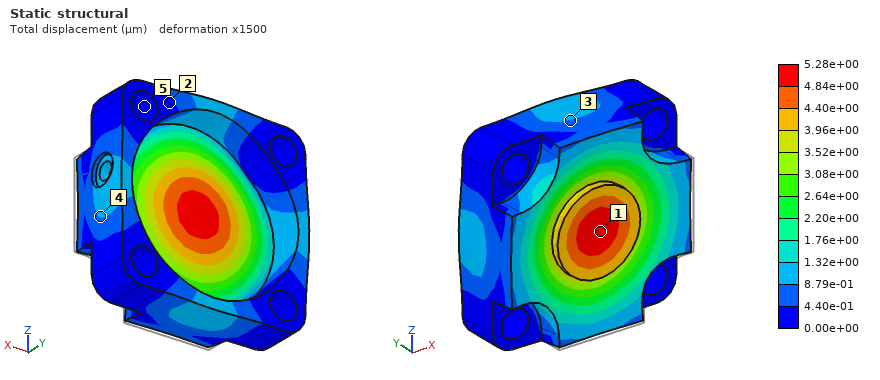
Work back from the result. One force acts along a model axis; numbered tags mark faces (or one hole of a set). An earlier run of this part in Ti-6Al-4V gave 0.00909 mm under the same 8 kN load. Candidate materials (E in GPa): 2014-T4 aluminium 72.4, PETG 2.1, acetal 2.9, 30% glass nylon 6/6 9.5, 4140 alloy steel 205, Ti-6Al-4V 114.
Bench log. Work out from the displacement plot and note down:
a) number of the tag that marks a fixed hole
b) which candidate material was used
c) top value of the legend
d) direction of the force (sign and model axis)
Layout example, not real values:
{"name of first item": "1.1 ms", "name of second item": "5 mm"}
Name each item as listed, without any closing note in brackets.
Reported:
{"number of the tag that marks a fixed hole": "5", "which candidate material was used": "4140 alloy steel", "top value of the legend": "5.28e+00 µm", "direction of the force": "+Y"}
